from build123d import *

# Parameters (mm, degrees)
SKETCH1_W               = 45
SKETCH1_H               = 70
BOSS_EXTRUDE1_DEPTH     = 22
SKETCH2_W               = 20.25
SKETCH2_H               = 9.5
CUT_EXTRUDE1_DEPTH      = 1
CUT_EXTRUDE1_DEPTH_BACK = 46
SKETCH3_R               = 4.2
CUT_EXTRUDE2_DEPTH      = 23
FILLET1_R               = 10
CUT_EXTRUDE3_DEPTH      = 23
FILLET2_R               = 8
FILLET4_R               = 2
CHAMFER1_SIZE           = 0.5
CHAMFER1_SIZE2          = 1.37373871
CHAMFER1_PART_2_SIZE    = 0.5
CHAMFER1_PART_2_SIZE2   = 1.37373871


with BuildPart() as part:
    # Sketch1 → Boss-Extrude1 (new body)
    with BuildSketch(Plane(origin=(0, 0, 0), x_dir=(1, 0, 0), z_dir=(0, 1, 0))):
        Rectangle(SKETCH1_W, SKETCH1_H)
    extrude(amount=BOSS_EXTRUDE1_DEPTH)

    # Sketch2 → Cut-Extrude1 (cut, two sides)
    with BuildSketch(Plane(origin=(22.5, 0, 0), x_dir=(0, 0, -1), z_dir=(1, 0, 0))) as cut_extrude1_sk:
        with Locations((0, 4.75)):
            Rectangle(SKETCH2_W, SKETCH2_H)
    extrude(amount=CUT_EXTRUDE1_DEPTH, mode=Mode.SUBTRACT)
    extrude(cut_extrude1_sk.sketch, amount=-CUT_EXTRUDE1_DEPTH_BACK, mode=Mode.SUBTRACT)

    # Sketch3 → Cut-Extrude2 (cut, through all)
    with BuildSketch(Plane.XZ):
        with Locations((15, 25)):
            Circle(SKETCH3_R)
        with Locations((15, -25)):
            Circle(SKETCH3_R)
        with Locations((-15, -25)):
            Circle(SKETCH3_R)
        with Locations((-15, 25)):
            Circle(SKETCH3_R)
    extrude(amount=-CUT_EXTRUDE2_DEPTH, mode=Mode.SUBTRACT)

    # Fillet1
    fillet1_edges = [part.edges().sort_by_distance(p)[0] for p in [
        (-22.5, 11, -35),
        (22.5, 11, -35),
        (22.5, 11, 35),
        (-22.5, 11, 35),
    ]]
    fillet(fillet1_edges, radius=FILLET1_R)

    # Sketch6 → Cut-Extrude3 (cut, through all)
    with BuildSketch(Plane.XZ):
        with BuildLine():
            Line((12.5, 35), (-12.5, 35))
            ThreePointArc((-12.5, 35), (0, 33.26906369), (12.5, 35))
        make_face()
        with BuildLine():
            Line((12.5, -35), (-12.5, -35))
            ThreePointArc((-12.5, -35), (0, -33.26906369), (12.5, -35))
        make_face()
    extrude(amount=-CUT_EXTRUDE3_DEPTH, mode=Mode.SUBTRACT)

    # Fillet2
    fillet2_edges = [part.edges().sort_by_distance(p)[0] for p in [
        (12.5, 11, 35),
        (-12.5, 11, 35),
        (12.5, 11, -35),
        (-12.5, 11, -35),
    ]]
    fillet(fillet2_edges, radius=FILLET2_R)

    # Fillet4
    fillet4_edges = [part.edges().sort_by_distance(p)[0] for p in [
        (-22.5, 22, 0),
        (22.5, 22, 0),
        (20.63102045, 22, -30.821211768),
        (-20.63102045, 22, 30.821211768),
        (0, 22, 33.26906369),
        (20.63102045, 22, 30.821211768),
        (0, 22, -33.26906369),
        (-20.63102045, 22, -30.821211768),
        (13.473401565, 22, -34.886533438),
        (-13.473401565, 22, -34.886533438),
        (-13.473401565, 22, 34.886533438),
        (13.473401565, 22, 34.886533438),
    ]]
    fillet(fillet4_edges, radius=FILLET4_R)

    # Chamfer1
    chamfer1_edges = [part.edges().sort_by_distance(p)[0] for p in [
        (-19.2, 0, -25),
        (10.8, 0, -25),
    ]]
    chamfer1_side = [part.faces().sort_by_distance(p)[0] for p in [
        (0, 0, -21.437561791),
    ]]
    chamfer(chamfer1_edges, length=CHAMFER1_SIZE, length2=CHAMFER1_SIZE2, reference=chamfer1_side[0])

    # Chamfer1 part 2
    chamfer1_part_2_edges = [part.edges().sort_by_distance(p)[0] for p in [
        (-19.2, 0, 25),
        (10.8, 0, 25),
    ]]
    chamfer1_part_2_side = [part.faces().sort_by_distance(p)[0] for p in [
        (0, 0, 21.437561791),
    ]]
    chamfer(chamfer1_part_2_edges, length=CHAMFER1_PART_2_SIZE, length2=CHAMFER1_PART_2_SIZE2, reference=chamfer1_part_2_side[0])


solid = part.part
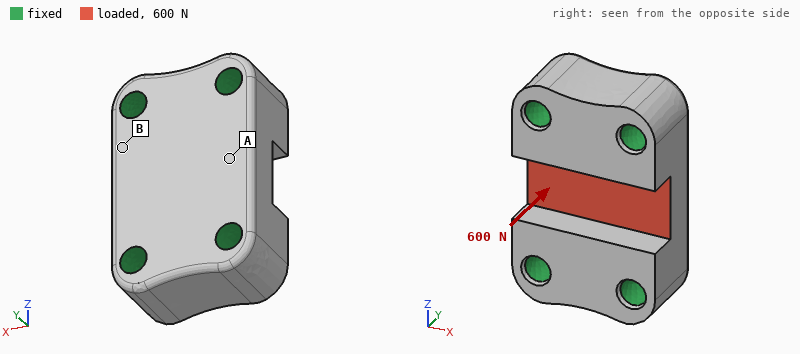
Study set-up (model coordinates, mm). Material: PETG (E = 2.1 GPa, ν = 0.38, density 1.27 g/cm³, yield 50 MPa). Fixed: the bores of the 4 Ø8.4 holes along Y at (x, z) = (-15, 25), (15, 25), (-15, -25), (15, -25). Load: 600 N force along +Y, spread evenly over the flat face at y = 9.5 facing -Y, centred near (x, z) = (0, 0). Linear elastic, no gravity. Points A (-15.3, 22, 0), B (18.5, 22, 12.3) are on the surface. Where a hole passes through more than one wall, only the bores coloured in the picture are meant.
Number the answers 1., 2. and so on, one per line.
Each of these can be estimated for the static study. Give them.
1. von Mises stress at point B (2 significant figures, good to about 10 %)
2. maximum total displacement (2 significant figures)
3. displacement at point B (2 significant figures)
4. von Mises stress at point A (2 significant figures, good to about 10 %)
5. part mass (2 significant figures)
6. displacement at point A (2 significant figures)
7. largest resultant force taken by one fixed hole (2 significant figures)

1. 0.31 MPa
2. 20 µm
3. 9.3 µm
4. 1.3 MPa
5. 67 g
6. 16 µm
7. 160 N
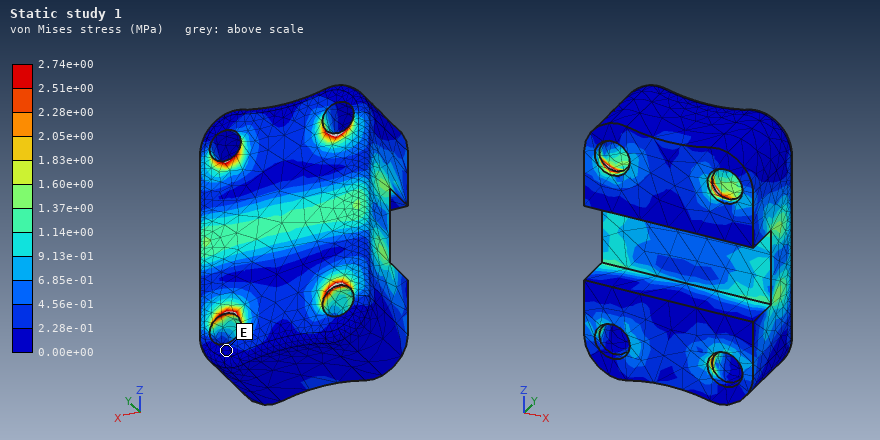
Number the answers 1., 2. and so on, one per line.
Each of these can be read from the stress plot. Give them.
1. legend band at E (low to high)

1. 0.00e+00 to 2.28e-01 MPa
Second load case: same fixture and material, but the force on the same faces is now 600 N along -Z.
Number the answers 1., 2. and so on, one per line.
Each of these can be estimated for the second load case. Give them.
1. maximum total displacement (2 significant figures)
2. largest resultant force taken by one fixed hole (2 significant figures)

1. 8.6 µm
2. 160 N
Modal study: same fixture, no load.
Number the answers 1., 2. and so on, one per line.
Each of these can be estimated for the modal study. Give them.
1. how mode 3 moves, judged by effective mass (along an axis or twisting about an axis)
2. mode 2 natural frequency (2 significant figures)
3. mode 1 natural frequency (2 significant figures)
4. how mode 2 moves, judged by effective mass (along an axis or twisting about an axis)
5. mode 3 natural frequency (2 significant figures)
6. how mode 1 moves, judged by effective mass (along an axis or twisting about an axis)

1. along X
2. 8000 Hz
3. 6900 Hz
4. along X
5. 8900 Hz
6. along Y
